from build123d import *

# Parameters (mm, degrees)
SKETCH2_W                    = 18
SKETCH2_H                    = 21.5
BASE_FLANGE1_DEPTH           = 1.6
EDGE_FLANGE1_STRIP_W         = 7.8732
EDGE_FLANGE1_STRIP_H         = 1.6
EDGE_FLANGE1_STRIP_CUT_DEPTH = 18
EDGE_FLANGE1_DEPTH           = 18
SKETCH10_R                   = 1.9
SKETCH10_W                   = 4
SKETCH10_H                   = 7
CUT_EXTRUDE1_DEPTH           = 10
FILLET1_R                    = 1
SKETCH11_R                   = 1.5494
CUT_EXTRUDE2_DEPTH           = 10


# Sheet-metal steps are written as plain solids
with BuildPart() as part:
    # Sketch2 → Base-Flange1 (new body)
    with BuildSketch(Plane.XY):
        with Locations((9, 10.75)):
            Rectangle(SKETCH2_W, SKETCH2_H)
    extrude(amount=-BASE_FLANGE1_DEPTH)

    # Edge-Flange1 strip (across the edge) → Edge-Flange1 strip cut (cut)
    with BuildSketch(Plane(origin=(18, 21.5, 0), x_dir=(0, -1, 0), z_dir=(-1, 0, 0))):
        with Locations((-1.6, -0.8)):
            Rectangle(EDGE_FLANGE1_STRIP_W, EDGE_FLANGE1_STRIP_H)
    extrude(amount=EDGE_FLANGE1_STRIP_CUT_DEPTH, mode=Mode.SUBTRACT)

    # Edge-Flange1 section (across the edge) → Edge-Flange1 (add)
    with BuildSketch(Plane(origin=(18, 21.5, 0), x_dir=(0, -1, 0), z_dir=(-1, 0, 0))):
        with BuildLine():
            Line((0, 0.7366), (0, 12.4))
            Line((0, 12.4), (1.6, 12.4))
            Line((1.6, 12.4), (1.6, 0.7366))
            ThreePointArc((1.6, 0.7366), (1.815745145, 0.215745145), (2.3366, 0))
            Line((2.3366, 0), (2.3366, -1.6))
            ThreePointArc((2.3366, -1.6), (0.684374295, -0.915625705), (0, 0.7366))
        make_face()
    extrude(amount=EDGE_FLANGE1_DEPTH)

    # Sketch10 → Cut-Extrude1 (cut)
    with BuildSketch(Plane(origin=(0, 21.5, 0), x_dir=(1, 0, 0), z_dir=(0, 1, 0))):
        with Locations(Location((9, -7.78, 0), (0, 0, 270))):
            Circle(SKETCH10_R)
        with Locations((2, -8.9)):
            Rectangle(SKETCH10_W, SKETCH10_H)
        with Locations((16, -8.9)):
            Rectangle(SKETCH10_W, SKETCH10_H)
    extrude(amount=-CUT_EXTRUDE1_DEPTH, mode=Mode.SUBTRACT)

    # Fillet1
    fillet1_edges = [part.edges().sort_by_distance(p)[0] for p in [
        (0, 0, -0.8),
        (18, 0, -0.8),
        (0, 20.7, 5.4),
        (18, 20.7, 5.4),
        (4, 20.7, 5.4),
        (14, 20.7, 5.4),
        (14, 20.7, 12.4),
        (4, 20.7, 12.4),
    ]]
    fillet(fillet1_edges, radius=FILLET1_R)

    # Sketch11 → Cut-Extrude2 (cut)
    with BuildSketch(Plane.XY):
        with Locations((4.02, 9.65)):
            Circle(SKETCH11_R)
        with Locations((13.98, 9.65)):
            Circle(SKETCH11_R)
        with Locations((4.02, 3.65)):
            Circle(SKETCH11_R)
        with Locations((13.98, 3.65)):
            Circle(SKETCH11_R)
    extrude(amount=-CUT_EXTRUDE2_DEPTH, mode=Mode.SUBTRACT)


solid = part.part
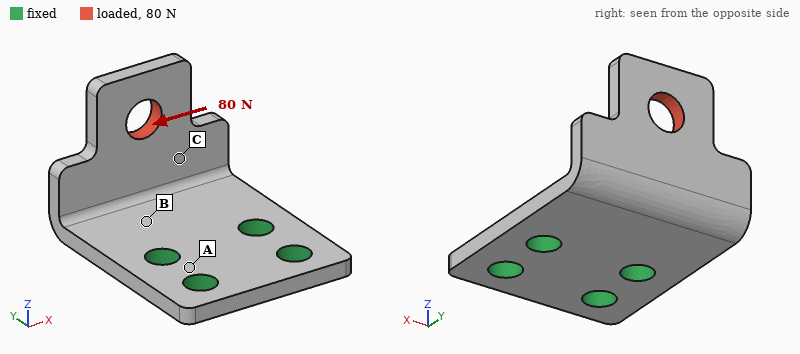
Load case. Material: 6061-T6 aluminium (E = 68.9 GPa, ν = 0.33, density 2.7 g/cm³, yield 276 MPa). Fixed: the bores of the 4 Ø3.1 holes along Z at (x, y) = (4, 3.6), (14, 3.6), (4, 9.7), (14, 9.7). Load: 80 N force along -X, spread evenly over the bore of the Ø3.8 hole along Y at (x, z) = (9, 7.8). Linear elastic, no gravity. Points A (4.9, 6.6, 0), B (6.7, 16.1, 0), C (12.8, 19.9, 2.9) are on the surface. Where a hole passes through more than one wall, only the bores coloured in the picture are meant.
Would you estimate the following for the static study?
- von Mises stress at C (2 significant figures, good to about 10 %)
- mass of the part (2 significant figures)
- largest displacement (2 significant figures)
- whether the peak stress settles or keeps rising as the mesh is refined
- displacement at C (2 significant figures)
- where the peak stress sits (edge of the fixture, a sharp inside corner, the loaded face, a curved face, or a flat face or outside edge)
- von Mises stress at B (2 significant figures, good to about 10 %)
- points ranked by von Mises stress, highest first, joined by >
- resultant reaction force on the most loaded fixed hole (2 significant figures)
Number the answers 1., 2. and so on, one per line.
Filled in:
1. 28 MPa
2. 2.2 g
3. 79 µm
4. keeps rising
5. 29 µm
6. edge of the fixture
7. 53 MPa
8. B > C > A
9. 94 N
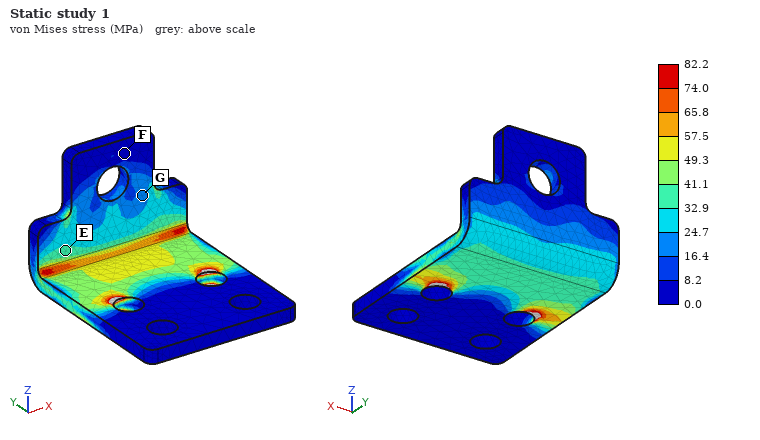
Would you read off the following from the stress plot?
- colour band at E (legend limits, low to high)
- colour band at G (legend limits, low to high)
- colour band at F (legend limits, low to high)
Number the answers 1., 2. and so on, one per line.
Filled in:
1. 32.9 to 41.1 MPa
2. 16.4 to 24.7 MPa
3. 0.0 to 8.2 MPa
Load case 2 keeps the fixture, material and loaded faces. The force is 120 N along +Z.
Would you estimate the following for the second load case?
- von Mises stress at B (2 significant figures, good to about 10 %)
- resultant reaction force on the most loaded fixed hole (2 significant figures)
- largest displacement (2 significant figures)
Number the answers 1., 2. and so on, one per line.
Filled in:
1. 65 MPa
2. 72 N
3. 0.21 mm
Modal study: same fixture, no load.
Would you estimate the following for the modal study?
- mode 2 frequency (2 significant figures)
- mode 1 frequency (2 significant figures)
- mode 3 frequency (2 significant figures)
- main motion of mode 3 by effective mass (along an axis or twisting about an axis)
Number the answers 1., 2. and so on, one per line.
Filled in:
1. 7700 Hz
2. 4200 Hz
3. 11 kHz
4. along Z
